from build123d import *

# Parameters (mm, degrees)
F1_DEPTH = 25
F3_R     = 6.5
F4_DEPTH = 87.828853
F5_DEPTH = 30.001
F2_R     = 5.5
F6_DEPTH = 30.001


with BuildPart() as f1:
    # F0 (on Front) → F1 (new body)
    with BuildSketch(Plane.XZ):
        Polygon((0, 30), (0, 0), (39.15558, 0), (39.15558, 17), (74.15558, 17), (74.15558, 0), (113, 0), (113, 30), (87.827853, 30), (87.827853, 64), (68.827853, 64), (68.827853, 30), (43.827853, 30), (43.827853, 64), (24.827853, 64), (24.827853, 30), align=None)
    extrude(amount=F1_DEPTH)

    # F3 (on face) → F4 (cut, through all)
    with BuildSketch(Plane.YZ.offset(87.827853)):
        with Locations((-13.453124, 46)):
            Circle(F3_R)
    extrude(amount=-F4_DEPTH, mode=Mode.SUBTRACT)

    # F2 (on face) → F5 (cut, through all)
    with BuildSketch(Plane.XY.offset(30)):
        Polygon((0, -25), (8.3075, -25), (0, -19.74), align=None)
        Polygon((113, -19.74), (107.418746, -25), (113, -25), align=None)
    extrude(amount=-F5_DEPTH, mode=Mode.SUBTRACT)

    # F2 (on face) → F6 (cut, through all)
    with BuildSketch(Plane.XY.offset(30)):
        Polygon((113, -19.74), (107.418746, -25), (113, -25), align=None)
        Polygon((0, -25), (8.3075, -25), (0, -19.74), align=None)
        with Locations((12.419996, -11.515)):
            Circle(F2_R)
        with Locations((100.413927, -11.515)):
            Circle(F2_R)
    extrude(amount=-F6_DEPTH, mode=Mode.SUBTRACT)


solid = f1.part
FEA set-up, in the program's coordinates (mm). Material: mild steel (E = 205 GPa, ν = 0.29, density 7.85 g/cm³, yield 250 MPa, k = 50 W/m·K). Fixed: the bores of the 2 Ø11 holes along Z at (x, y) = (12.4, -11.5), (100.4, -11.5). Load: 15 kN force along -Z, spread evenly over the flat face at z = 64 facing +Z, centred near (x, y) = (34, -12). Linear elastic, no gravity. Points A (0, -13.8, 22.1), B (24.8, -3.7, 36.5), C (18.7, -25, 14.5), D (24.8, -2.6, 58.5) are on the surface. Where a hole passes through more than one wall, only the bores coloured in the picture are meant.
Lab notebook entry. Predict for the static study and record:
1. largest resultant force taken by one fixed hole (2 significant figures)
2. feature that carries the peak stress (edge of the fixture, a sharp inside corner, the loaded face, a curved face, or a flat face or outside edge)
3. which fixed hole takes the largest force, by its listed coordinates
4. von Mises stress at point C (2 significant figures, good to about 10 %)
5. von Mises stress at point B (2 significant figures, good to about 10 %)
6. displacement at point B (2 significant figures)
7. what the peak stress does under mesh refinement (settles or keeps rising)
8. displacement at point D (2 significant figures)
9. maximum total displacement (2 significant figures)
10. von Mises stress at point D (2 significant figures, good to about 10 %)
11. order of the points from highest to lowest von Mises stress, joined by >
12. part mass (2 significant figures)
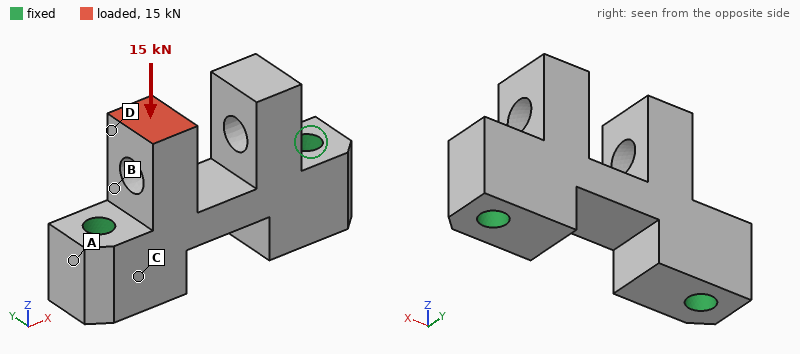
14 kN
edge of the fixture
(12.4, -11.5)
22 MPa
51 MPa
7.1 µm
keeps rising
14 µm
23 µm
41 MPa
B > D > C > A
710 g
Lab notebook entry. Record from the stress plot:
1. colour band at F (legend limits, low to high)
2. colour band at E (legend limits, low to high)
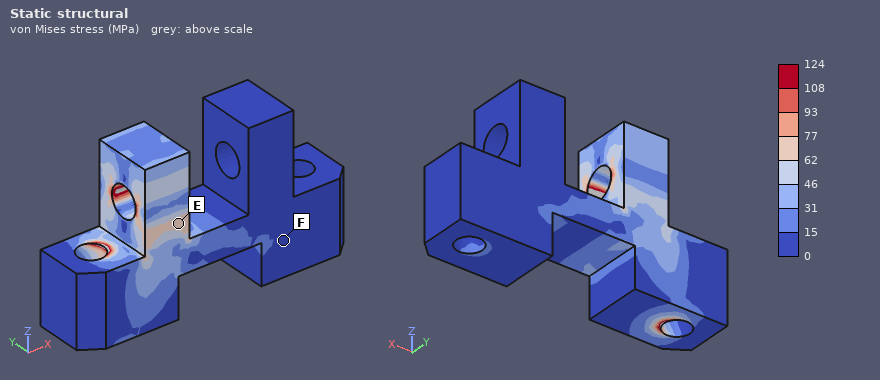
0 to 15 MPa
62 to 77 MPa
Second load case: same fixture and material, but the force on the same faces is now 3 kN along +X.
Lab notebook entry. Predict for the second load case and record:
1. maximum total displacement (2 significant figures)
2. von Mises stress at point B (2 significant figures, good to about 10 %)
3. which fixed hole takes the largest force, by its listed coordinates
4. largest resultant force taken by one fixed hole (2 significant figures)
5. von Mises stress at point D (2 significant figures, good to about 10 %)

43 µm
77 MPa
(100.4, -11.5)
2.1 kN
16 MPa
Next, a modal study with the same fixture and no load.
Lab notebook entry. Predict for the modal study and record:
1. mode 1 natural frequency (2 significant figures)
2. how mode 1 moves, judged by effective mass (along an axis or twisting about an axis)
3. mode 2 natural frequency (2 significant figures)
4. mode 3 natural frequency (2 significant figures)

5800 Hz
along Y
6600 Hz
6700 Hz
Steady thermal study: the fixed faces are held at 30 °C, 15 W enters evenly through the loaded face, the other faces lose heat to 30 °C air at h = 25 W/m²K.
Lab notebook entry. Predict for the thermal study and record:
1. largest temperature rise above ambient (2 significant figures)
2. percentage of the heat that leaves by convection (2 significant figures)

36 K
17 %
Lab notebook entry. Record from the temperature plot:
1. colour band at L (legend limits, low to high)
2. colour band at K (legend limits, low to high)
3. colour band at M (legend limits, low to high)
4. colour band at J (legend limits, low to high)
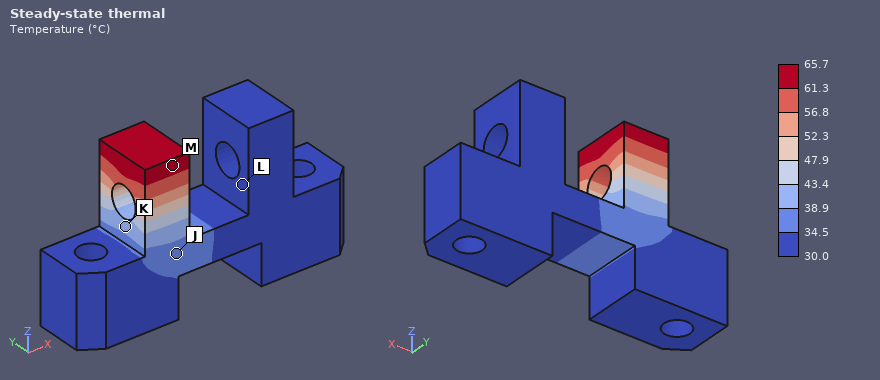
30.0 to 34.5 °C
38.9 to 43.4 °C
61.3 to 65.7 °C
34.5 to 38.9 °C
